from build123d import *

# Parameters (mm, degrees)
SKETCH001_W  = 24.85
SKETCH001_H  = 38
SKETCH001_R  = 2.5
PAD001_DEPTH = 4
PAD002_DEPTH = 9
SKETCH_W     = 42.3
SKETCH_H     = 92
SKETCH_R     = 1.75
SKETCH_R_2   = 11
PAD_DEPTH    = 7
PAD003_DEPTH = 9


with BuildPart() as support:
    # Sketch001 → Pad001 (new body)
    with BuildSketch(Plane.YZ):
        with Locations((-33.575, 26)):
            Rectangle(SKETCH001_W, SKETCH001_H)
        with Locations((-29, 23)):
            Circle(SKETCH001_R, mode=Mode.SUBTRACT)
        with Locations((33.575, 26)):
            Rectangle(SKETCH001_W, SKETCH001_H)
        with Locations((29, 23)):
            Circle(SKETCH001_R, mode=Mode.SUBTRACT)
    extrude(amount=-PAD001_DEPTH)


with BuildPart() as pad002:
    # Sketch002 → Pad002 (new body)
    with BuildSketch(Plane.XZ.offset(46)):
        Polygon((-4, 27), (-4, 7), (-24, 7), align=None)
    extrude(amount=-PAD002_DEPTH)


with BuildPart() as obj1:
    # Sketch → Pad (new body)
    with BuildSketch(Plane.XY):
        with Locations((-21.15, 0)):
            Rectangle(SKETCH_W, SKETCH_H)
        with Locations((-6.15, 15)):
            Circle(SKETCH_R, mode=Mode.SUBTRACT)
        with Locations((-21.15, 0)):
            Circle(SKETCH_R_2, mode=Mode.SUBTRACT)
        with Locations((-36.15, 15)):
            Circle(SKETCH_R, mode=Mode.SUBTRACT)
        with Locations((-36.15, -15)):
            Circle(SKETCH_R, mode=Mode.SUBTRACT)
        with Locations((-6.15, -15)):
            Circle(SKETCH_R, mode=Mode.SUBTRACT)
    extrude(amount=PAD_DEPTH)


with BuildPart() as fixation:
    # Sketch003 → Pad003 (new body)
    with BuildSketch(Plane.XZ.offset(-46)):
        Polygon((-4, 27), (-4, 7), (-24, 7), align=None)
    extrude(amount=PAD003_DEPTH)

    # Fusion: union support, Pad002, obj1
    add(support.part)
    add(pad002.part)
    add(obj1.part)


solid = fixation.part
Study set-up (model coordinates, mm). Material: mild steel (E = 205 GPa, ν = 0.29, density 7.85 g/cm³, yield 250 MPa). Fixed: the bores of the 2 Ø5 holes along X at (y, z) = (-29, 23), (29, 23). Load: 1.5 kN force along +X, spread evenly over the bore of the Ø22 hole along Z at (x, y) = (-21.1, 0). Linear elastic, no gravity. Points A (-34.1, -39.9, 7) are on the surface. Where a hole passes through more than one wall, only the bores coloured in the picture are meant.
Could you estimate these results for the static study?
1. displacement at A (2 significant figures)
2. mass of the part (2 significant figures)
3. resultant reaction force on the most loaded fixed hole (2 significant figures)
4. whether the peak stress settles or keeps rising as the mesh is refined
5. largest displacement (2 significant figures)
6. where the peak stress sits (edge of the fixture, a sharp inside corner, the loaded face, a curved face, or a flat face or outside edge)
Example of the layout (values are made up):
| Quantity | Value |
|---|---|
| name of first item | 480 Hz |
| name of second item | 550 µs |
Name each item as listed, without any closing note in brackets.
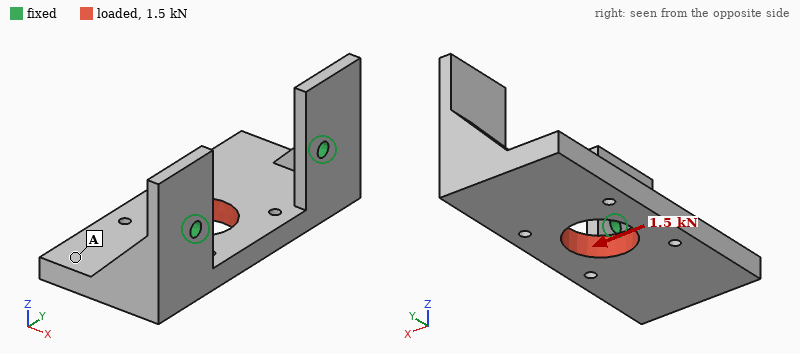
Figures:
| Quantity | Value |
|---|---|
| displacement at A | 0.083 mm |
| mass of the part | 280 g |
| resultant reaction force on the most loaded fixed hole | 750 N |
| whether the peak stress settles or keeps rising as the mesh is refined | keeps rising |
| largest displacement | 0.11 mm |
| where the peak stress sits | edge of the fixture |
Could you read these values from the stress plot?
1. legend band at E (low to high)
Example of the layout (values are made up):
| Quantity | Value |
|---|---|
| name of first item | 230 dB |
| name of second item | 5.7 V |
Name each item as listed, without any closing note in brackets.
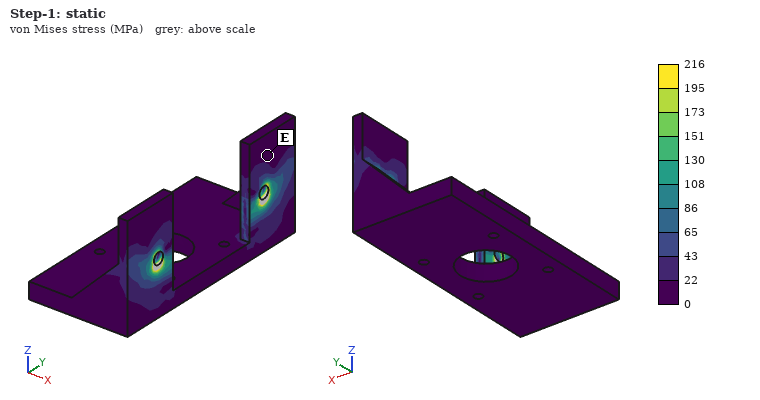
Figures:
| Quantity | Value |
|---|---|
| legend band at E | 0 to 22 MPa |
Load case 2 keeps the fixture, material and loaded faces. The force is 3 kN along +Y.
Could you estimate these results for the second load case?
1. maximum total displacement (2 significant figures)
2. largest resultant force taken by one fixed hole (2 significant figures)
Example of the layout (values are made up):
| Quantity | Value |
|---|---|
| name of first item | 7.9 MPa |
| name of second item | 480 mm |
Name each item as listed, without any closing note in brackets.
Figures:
| Quantity | Value |
|---|---|
| maximum total displacement | 60 µm |
| largest resultant force taken by one fixed hole | 1.8 kN |
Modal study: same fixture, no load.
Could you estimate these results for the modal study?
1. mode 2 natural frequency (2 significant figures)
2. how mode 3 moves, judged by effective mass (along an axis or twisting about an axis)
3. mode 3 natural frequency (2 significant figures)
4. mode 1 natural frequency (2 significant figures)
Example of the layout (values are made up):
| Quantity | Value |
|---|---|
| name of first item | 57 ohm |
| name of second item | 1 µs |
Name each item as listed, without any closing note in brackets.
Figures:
| Quantity | Value |
|---|---|
| mode 2 natural frequency | 2200 Hz |
| how mode 3 moves, judged by effective mass | along Y |
| mode 3 natural frequency | 3900 Hz |
| mode 1 natural frequency | 1200 Hz |
